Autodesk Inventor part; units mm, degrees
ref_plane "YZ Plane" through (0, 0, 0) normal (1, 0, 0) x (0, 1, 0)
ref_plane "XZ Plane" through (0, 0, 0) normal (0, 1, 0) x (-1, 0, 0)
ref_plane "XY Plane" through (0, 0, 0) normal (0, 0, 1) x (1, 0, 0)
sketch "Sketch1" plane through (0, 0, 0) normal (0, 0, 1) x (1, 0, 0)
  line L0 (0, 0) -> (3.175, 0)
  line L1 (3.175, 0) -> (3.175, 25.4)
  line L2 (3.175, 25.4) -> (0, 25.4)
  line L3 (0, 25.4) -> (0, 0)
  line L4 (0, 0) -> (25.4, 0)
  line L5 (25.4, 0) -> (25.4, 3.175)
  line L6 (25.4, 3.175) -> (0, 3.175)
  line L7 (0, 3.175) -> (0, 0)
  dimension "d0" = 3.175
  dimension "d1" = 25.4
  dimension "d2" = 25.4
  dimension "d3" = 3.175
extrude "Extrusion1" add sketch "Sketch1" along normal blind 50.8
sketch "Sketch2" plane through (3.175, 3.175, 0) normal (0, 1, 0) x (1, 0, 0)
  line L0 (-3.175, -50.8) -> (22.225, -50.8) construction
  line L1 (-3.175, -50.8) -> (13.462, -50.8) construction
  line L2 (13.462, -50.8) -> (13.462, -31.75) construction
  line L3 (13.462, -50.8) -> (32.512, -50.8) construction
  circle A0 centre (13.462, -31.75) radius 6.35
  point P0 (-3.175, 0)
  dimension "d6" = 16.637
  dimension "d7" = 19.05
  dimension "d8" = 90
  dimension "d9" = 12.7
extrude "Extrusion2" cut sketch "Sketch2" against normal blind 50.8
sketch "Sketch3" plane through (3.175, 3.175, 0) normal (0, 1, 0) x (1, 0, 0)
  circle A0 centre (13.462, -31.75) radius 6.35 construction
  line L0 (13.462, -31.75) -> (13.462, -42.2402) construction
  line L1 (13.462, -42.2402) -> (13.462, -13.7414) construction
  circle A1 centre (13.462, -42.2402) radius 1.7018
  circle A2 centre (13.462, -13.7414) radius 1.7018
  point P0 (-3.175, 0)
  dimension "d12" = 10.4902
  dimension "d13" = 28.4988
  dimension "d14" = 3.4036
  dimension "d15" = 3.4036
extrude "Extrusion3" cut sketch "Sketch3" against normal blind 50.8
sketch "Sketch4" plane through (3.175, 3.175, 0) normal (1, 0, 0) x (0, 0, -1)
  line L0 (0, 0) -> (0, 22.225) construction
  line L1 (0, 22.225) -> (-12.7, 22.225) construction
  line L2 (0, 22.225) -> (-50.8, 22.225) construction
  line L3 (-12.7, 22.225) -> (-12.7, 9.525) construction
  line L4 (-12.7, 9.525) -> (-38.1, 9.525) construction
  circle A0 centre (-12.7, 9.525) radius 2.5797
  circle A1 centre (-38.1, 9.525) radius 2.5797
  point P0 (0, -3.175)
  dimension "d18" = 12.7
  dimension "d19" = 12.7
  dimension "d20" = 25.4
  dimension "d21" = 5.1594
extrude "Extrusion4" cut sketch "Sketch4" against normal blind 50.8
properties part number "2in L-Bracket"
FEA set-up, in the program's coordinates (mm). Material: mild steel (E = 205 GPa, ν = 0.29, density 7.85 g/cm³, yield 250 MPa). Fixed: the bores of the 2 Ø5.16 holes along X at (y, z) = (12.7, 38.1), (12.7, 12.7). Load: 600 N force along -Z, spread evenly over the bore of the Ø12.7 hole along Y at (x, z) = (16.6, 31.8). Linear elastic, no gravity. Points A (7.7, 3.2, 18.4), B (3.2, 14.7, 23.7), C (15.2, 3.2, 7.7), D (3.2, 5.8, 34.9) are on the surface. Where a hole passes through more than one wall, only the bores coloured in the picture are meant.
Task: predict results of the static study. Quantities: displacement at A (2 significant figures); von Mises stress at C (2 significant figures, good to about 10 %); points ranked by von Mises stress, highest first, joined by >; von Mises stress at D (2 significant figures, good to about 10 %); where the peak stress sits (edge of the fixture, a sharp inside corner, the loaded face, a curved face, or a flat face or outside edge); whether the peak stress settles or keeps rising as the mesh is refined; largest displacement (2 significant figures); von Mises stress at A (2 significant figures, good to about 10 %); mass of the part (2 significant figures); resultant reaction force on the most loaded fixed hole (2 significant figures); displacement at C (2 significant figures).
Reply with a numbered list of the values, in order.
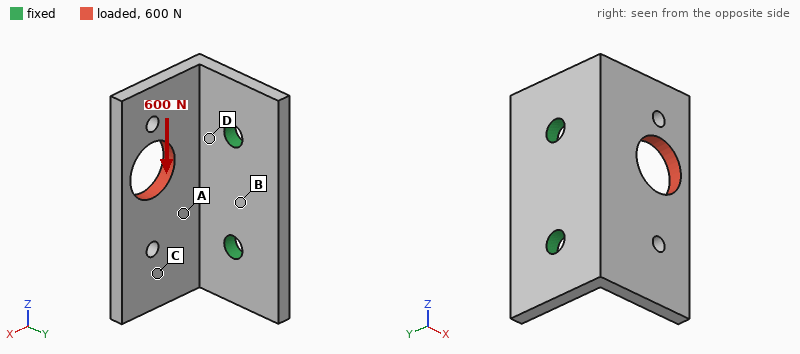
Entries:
1. 5.0 µm
2. 12 MPa
3. D > A > C > B
4. 34 MPa
5. edge of the fixture
6. keeps rising
7. 23 µm
8. 21 MPa
9. 56 g
10. 480 N
11. 13 µm
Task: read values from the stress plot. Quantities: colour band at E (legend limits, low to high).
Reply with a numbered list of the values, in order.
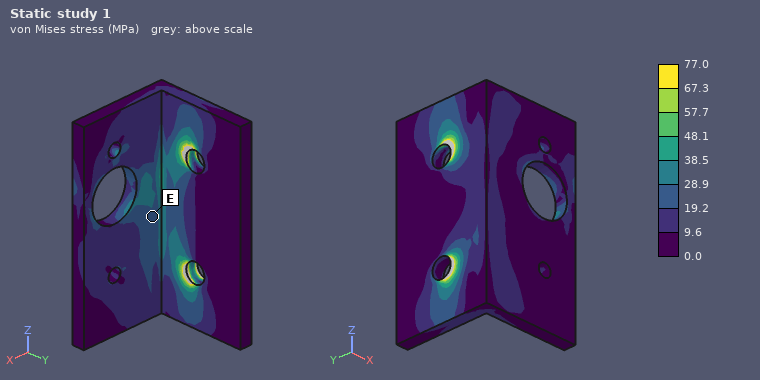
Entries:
1. 19.2 to 28.9 MPa
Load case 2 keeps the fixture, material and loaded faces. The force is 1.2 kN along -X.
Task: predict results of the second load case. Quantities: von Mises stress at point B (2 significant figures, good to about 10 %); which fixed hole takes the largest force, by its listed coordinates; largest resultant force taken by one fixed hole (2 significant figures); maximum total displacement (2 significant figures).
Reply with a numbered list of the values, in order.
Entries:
1. 30 MPa
2. (12.7, 38.1)
3. 850 N
4. 77 µm
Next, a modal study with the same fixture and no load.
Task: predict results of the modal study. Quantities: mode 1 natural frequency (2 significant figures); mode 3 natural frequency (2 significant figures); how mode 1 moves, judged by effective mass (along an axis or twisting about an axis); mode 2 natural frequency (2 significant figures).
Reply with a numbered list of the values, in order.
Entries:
1. 2900 Hz
2. 7700 Hz
3. along Y
4. 4600 Hz
